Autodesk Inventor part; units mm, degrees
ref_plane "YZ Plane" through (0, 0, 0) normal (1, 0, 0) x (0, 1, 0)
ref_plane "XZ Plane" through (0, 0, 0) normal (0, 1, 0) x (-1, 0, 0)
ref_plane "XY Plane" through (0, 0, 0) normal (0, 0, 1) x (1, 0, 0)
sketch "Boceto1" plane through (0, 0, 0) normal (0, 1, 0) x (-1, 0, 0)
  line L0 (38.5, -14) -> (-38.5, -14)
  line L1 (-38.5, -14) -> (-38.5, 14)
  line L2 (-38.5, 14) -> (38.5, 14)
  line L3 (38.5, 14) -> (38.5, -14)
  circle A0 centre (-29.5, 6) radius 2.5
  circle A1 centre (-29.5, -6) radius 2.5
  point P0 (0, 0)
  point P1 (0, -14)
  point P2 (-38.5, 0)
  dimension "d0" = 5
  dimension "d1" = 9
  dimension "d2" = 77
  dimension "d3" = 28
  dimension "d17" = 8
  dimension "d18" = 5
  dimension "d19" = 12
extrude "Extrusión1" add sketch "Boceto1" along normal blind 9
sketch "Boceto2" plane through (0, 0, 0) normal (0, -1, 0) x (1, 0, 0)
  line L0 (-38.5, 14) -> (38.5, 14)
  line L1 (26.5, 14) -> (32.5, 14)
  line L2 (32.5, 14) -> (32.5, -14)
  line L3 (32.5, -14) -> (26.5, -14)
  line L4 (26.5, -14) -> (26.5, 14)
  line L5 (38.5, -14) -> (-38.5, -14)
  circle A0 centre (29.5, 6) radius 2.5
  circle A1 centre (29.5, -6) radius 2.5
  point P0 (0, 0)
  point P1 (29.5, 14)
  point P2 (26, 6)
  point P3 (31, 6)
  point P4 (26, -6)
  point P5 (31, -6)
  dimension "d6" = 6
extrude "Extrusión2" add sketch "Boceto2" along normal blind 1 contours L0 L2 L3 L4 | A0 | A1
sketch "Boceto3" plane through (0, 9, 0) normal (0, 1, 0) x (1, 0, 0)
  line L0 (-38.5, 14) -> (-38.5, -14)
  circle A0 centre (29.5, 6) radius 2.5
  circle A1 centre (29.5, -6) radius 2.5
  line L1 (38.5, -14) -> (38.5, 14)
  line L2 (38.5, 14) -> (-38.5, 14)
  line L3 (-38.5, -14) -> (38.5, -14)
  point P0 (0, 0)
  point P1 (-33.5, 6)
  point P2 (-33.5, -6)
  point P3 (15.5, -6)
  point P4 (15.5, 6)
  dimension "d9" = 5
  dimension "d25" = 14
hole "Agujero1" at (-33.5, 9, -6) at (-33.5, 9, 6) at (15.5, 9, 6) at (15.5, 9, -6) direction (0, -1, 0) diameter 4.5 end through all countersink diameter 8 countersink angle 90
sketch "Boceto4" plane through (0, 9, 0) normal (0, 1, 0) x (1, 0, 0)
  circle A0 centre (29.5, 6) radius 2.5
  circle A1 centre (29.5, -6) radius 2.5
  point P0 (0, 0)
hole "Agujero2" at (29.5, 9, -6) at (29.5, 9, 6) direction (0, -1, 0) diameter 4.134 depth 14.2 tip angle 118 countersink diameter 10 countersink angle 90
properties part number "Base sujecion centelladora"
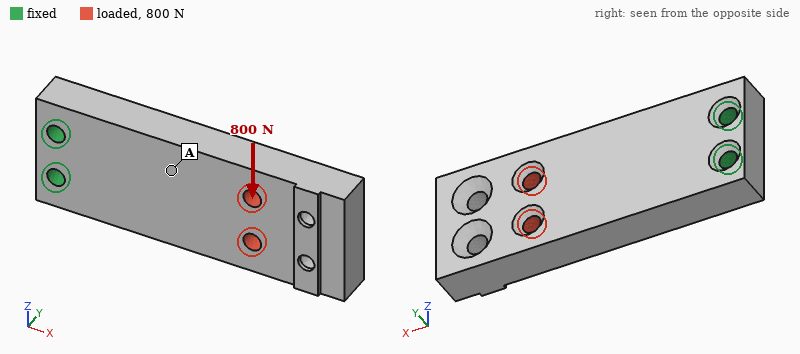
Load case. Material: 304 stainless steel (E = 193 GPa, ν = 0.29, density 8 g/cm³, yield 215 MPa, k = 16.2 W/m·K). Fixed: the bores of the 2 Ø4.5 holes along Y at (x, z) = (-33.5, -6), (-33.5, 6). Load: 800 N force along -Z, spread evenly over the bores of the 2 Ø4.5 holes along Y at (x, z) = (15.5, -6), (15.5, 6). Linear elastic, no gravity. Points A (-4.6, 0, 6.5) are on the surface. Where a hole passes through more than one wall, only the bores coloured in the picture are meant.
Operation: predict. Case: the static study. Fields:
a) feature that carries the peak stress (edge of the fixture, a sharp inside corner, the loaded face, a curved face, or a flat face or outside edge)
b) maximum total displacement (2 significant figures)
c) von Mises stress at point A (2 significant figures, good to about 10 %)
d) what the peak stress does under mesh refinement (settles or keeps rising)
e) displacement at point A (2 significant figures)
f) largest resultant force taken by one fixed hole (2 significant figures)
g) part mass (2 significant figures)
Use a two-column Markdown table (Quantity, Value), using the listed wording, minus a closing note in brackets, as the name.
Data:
| Quantity | Value |
|---|---|
| feature that carries the peak stress | edge of the fixture |
| maximum total displacement | 26 µm |
| von Mises stress at point A | 11 MPa |
| what the peak stress does under mesh refinement | keeps rising |
| displacement at point A | 8.2 µm |
| largest resultant force taken by one fixed hole | 2.5 kN |
| part mass | 150 g |
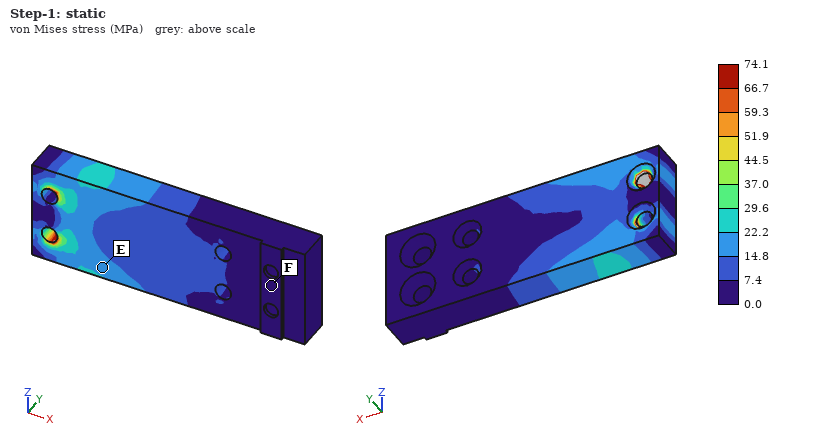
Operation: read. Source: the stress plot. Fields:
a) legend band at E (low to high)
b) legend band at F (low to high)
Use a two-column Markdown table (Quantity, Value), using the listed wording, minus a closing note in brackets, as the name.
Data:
| Quantity | Value |
|---|---|
| legend band at E | 14.8 to 22.2 MPa |
| legend band at F | 0.0 to 7.4 MPa |
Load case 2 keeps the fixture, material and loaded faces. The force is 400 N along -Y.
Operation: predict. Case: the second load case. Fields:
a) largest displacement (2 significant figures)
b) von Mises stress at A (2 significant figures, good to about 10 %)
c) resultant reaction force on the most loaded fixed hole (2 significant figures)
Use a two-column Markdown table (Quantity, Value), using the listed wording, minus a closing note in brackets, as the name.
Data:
| Quantity | Value |
|---|---|
| largest displacement | 88 µm |
| von Mises stress at A | 21 MPa |
| resultant reaction force on the most loaded fixed hole | 200 N |
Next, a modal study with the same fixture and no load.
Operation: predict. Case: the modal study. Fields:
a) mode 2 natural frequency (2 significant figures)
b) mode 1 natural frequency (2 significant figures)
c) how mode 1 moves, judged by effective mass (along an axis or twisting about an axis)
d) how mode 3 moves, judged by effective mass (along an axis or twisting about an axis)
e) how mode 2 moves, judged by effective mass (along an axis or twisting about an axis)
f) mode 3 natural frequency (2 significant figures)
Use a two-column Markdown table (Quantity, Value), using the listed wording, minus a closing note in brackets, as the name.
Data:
| Quantity | Value |
|---|---|
| mode 2 natural frequency | 3500 Hz |
| mode 1 natural frequency | 1400 Hz |
| how mode 1 moves, judged by effective mass | along Y |
| how mode 3 moves, judged by effective mass | twisting about X |
| how mode 2 moves, judged by effective mass | along Z |
| mode 3 natural frequency | 6100 Hz |
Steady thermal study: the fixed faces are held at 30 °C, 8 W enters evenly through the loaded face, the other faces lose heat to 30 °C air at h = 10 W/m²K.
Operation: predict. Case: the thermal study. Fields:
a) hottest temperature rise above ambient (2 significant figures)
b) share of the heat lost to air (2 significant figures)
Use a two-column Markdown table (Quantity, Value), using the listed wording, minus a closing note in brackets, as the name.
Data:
| Quantity | Value |
|---|---|
| hottest temperature rise above ambient | 74 K |
| share of the heat lost to air | 33 % |
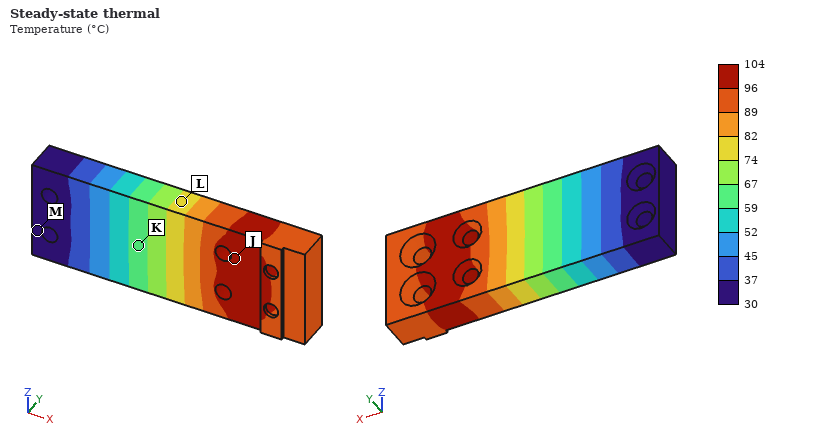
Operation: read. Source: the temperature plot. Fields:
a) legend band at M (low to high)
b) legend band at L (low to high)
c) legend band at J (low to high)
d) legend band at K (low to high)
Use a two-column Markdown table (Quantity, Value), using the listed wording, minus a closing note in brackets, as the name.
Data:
| Quantity | Value |
|---|---|
| legend band at M | 30 to 37 °C |
| legend band at L | 74 to 82 °C |
| legend band at J | 96 to 104 °C |
| legend band at K | 59 to 67 °C |
